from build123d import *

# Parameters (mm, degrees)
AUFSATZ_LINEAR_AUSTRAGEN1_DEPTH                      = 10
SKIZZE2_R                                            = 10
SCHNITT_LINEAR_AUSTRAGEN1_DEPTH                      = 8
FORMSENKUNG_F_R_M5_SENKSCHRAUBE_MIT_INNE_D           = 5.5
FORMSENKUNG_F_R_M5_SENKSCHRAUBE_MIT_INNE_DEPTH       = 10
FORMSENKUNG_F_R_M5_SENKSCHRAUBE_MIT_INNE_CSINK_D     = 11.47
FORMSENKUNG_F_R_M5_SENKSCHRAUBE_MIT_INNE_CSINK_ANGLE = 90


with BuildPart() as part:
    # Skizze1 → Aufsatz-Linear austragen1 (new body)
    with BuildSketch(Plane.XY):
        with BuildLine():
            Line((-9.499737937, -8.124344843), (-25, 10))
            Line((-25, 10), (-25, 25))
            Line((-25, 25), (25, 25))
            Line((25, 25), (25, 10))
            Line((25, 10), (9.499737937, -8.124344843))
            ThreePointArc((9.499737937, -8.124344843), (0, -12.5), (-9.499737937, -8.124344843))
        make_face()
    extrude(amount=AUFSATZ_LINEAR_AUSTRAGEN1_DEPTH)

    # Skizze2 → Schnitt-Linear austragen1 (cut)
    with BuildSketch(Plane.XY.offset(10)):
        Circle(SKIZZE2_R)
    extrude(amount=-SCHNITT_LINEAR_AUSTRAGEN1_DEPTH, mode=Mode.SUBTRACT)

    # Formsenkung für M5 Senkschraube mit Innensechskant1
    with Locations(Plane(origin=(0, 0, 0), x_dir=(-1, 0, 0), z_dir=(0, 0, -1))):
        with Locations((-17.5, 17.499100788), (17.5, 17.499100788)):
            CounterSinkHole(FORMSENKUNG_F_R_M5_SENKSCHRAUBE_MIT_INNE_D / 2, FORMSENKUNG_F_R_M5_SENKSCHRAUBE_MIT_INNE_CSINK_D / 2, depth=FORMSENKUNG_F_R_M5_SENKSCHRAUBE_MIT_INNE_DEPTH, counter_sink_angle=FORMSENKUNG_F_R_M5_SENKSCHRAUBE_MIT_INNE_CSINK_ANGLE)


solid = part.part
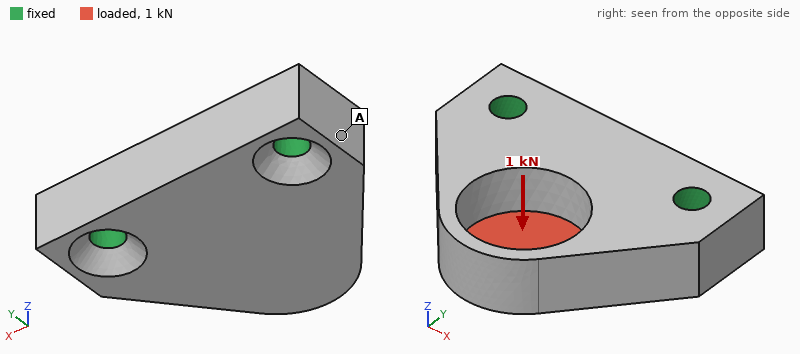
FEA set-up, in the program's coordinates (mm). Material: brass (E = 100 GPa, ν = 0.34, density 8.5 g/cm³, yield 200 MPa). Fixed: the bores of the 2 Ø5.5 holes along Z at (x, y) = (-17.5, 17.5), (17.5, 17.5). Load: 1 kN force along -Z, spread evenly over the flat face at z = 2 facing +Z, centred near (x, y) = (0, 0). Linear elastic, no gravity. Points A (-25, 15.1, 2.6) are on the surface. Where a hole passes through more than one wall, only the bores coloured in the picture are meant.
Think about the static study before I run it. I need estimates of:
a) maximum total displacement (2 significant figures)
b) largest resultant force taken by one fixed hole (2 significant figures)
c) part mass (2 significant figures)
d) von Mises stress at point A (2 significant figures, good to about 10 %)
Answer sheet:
33 µm
530 N
95 g
11 MPa
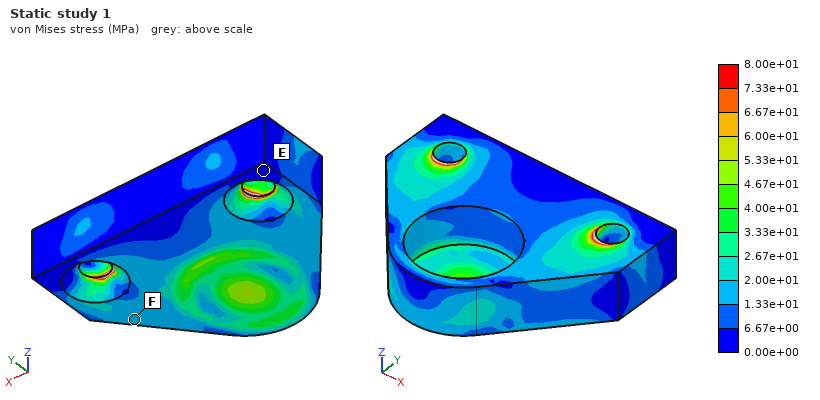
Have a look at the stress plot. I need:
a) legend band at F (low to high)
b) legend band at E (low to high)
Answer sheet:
1.33e+01 to 2.00e+01 MPa
0.00e+00 to 6.67e+00 MPa
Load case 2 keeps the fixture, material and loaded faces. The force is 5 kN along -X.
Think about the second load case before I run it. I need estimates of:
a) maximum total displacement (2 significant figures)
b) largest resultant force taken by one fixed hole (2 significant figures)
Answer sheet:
21 µm
3.4 kN
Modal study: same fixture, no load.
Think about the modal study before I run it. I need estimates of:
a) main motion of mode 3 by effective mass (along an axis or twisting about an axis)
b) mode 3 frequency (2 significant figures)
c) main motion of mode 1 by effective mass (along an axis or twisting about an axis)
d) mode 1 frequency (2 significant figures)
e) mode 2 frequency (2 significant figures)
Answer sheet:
along Z
19 kHz
along Z
6900 Hz
13 kHz
